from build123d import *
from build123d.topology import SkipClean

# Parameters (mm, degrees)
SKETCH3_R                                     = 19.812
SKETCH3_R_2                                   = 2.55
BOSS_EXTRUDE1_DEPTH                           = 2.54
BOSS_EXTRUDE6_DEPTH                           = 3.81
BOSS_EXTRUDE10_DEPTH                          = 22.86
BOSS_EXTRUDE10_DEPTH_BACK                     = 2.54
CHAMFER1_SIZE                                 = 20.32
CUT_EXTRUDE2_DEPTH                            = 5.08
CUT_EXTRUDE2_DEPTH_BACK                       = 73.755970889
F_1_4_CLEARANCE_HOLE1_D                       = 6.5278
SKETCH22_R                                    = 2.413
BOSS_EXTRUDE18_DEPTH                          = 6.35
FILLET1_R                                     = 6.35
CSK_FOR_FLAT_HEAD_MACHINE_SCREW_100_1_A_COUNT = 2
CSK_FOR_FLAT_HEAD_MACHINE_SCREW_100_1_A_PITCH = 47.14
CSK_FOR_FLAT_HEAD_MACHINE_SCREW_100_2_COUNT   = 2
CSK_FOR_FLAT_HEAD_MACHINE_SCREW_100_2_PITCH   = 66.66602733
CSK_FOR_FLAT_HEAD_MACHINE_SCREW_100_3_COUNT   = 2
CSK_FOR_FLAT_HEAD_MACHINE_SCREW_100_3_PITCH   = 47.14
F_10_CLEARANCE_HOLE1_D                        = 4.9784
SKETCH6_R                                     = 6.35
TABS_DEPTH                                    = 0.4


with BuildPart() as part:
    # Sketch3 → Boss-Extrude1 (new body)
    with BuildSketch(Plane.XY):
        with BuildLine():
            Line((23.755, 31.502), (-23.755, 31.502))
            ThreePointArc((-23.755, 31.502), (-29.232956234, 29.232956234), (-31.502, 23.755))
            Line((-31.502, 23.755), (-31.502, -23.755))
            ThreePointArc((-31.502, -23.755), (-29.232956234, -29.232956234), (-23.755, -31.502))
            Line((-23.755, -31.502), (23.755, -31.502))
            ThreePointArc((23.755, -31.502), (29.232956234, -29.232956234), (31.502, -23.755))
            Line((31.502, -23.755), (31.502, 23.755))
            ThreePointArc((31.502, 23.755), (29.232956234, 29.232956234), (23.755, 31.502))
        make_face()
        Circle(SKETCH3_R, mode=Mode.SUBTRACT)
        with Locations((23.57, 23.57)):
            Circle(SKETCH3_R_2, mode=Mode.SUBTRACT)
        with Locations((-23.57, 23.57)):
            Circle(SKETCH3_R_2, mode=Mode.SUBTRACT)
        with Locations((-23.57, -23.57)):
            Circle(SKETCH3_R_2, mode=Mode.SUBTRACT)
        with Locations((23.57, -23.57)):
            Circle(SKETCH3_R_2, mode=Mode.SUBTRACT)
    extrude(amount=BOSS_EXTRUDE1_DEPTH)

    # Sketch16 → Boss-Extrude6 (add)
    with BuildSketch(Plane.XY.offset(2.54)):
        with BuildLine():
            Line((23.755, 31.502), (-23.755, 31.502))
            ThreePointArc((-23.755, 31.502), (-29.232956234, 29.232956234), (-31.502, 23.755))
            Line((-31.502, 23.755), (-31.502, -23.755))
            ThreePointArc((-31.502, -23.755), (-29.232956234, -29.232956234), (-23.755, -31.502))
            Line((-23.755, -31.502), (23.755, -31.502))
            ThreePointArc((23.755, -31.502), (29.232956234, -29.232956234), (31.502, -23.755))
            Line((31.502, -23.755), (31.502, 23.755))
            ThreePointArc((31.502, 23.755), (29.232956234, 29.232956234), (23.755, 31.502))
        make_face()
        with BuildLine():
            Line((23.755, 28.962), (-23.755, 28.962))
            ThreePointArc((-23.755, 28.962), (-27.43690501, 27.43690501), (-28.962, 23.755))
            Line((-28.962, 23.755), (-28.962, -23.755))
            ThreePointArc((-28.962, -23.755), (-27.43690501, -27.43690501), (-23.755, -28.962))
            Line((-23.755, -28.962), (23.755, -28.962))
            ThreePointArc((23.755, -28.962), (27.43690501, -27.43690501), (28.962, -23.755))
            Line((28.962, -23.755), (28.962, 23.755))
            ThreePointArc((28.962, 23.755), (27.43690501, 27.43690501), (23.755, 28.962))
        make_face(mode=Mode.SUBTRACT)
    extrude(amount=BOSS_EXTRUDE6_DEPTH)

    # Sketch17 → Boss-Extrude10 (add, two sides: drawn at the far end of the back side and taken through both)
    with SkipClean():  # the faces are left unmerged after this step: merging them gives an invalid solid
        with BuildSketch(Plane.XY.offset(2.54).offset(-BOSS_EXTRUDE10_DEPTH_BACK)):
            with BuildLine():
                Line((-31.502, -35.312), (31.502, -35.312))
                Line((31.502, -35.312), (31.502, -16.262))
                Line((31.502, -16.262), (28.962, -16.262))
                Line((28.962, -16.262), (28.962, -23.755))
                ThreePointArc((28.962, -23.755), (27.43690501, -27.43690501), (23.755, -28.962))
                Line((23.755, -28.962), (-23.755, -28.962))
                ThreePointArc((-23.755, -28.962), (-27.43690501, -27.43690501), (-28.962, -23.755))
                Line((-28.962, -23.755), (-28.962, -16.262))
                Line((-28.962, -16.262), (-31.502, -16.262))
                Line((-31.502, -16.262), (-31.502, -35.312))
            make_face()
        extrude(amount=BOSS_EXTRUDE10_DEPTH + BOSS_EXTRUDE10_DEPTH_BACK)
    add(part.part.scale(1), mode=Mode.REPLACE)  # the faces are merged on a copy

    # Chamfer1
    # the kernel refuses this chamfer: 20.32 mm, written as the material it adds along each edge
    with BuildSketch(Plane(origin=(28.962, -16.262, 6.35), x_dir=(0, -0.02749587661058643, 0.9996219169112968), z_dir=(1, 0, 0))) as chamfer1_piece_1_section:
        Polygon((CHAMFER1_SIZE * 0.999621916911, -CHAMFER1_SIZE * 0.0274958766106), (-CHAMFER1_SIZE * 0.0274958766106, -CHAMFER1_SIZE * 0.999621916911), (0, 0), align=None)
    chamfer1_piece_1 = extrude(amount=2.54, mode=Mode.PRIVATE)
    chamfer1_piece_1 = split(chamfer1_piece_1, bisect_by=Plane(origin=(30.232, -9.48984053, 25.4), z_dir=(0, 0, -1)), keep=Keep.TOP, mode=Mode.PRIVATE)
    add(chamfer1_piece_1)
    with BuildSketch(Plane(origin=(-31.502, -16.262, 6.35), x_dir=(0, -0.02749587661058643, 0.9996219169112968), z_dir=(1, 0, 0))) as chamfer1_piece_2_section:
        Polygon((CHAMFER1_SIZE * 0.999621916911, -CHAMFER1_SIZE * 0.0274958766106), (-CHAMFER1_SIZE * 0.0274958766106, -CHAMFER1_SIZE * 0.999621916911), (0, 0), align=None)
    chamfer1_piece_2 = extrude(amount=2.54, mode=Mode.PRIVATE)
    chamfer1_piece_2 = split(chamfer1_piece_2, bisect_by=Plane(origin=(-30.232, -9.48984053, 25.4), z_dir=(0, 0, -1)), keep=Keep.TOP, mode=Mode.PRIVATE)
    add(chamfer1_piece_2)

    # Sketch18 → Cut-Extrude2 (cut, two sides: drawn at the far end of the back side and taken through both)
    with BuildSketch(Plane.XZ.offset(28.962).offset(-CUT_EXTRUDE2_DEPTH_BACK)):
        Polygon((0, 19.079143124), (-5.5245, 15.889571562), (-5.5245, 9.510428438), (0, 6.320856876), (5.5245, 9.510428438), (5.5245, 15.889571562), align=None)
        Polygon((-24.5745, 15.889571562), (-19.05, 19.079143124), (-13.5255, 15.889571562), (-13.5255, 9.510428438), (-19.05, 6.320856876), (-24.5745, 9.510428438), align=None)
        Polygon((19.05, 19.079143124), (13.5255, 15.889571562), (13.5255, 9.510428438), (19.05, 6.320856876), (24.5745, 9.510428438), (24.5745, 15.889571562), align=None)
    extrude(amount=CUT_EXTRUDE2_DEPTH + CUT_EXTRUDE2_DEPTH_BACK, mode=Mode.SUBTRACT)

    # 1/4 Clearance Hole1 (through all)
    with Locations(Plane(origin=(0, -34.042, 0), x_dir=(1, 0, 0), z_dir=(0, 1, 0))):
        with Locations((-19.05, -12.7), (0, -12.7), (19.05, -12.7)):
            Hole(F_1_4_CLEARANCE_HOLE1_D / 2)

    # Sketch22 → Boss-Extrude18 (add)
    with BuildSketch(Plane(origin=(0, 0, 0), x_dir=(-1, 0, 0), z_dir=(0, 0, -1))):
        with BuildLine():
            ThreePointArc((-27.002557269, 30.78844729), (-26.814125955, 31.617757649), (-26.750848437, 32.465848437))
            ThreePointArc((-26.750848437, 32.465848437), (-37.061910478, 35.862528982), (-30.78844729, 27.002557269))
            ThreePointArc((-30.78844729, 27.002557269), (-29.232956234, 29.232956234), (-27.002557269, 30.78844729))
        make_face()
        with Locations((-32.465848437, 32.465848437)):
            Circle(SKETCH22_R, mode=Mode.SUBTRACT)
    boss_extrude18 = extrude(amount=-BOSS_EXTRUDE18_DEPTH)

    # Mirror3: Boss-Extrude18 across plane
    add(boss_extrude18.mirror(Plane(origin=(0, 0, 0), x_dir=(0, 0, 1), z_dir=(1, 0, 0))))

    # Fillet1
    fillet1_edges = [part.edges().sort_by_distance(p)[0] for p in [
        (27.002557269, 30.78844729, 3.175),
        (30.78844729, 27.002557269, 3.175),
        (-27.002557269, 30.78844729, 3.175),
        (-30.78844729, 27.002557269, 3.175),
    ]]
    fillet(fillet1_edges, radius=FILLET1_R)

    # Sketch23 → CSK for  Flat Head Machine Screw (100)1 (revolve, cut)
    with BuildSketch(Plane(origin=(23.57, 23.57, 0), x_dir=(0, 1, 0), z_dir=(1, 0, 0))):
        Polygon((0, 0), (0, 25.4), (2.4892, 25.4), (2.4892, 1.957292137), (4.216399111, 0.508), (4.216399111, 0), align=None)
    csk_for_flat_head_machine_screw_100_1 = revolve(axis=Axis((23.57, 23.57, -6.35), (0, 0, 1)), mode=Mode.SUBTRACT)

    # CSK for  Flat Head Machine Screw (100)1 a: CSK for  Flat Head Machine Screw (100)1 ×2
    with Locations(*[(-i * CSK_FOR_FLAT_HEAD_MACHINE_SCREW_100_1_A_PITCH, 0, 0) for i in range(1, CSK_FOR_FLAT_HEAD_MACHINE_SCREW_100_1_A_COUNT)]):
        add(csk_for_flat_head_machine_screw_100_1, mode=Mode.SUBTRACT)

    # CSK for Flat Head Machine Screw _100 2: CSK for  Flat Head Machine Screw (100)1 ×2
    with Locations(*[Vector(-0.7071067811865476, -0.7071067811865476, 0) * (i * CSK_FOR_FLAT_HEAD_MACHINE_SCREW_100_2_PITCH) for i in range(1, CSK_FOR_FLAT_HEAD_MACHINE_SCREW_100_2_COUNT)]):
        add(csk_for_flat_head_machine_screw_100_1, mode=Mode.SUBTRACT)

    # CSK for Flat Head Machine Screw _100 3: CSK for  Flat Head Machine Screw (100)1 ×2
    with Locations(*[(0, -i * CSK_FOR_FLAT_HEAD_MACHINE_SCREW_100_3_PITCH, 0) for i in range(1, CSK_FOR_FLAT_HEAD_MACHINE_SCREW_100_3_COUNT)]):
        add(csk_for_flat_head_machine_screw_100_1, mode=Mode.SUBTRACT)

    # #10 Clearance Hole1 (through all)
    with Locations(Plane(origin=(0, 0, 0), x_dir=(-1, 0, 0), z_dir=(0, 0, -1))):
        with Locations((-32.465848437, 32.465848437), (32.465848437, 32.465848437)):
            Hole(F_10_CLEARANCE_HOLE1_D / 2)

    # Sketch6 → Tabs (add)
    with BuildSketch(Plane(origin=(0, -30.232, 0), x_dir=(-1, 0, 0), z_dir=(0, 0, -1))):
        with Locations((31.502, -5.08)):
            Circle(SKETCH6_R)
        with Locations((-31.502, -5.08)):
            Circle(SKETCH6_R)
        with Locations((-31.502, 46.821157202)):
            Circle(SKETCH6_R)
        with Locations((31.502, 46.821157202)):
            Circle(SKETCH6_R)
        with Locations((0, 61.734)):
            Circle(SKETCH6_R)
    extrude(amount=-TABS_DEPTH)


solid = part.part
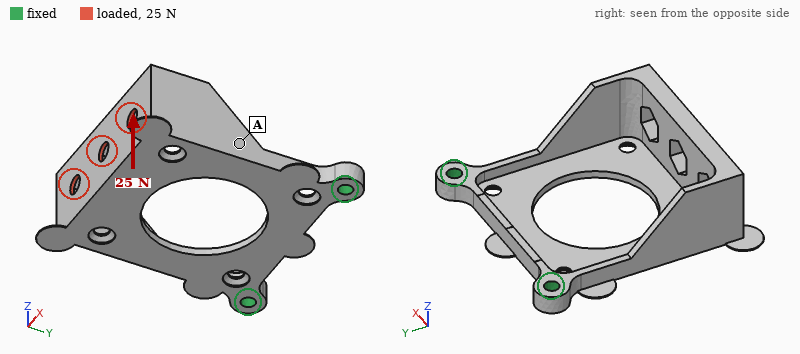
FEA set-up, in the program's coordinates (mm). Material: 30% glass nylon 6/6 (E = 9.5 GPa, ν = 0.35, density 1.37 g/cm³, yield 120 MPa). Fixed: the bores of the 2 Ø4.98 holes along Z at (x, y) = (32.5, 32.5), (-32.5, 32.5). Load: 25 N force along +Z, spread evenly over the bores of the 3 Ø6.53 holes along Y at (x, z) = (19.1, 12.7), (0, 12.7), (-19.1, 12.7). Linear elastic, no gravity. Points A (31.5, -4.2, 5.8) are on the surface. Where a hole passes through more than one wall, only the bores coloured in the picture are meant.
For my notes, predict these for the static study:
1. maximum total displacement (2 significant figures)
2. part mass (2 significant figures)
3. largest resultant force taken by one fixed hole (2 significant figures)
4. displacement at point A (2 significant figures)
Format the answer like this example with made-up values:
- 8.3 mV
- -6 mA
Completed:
- 1.1 mm
- 27 g
- 29 N
- 0.41 mm
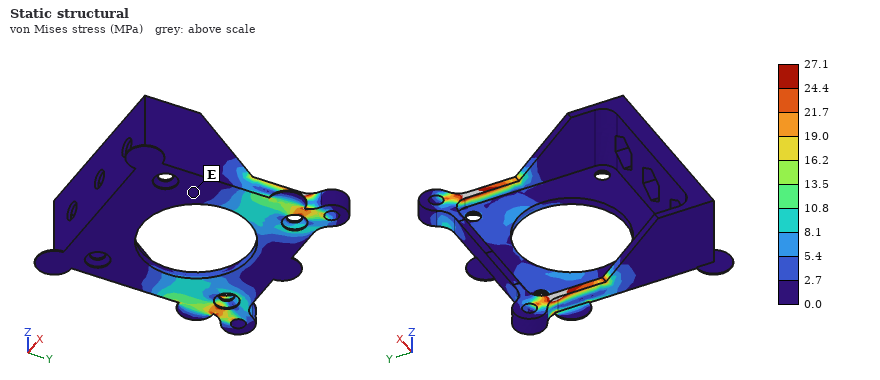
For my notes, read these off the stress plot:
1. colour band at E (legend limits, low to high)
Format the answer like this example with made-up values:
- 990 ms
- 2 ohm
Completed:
- 0.0 to 2.7 MPa
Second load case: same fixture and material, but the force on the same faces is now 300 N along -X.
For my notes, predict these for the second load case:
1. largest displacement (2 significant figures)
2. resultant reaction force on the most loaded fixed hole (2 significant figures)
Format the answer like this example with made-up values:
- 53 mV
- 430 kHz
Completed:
- 1.3 mm
- 350 N
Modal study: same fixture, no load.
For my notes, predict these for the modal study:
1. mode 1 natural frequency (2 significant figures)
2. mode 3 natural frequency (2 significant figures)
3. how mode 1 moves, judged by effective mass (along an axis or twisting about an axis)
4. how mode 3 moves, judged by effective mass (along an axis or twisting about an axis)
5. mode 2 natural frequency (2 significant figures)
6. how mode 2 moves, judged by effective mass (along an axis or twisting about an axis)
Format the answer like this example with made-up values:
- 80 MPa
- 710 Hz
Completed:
- 200 Hz
- 1600 Hz
- along Z
- along X
- 560 Hz
- along X
